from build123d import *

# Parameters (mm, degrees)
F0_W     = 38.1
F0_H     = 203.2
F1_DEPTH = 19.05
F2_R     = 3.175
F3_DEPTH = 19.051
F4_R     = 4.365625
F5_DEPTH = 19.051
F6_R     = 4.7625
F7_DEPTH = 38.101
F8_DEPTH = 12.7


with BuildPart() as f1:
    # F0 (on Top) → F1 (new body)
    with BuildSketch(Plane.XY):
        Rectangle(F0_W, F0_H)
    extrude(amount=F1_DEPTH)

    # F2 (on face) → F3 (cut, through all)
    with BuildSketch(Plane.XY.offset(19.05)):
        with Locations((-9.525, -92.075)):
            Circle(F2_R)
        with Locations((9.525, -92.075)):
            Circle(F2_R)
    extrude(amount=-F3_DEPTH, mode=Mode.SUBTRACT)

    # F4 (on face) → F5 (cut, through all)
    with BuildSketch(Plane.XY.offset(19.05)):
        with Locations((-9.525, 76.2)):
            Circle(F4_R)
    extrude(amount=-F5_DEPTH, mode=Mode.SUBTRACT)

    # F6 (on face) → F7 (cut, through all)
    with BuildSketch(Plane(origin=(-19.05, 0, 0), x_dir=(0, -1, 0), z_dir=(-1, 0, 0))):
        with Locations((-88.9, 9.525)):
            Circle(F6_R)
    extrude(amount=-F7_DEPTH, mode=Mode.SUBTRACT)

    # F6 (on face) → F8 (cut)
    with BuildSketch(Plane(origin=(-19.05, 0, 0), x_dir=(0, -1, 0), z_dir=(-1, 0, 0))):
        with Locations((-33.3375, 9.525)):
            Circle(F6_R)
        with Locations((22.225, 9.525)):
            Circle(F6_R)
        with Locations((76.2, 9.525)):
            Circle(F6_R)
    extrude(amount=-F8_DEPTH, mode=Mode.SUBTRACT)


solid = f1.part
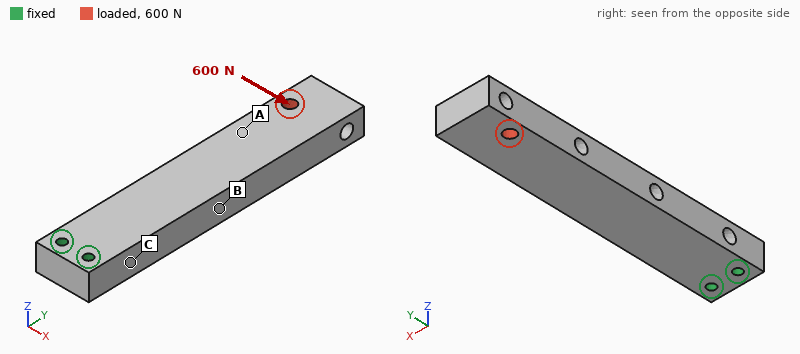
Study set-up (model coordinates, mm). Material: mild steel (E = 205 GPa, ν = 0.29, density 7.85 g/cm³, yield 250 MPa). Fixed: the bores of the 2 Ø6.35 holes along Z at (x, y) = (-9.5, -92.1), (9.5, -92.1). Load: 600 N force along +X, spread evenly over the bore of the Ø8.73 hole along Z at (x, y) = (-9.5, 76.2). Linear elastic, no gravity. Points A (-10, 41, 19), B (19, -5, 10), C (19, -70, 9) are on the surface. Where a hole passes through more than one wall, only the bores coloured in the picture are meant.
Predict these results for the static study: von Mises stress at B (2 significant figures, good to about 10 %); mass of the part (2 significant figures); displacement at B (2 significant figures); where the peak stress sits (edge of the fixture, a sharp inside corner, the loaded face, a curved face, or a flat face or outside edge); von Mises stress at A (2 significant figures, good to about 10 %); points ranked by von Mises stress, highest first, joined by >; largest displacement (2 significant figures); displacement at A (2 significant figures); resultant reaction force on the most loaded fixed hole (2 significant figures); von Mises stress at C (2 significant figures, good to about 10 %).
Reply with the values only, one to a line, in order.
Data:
11 MPa
1.1 kg
24 µm
a curved face
4.4 MPa
C > B > A
79 µm
46 µm
4.4 kN
21 MPa
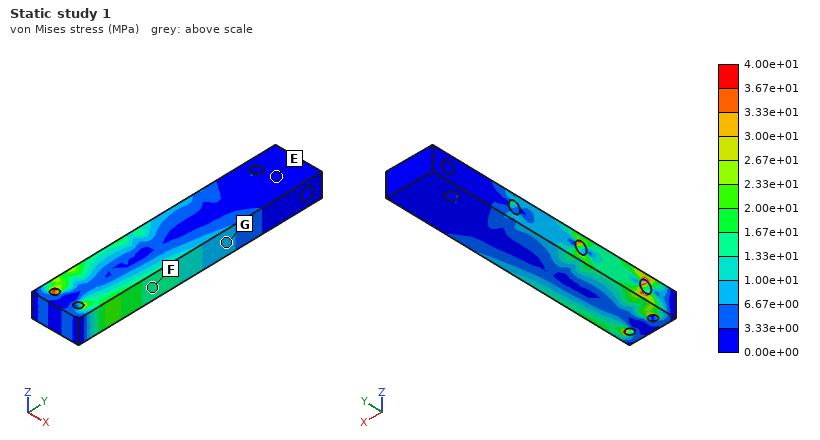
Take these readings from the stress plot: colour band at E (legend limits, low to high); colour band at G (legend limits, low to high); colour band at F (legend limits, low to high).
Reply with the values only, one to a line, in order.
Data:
0.00e+00 to 3.33e+00 MPa
6.67e+00 to 1.00e+01 MPa
1.33e+01 to 1.67e+01 MPa
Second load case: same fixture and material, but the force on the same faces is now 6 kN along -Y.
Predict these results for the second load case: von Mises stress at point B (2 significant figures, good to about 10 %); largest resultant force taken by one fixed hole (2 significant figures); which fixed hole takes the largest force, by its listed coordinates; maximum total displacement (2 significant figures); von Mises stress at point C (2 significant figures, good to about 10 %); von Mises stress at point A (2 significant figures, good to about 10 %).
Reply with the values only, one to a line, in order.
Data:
5.1 MPa
5.5 kN
(-9.5, -92.1)
77 µm
6.7 MPa
21 MPa
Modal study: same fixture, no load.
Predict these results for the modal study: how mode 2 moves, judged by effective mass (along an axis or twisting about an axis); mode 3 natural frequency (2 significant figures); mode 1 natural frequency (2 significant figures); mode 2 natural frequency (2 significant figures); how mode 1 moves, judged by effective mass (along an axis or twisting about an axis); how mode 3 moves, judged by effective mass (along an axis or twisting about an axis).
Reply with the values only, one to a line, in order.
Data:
along X
2600 Hz
440 Hz
790 Hz
along Z
along Z
